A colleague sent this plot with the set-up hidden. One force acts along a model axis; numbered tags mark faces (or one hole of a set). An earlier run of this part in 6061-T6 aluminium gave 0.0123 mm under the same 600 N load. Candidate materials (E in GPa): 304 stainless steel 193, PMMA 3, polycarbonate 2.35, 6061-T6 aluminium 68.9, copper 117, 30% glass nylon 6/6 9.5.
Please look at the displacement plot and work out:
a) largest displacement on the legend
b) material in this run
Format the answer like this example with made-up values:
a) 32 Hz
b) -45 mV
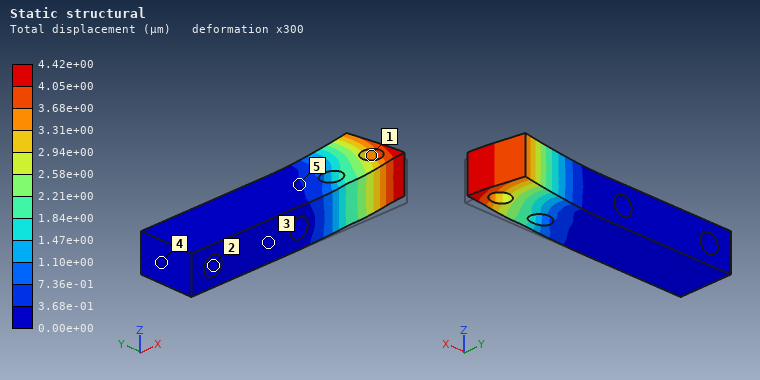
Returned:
a) 4.42e+00 µm
b) 304 stainless steel
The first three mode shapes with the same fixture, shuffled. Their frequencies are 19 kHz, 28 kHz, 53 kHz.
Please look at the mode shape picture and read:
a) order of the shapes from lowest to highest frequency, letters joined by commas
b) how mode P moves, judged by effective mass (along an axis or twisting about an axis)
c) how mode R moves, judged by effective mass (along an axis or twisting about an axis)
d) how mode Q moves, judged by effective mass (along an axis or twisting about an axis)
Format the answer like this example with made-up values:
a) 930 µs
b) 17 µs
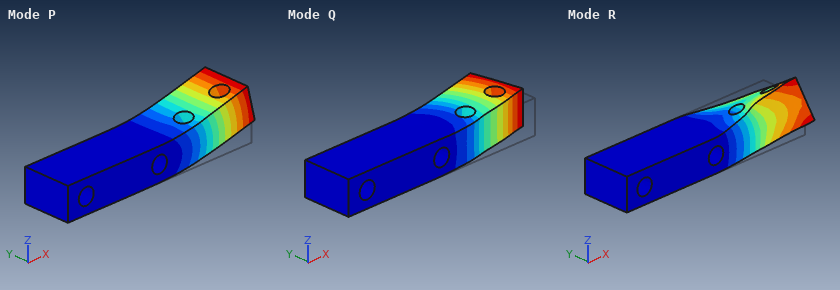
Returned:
a) P, Q, R
b) along Z
c) twisting about X
d) along Y
